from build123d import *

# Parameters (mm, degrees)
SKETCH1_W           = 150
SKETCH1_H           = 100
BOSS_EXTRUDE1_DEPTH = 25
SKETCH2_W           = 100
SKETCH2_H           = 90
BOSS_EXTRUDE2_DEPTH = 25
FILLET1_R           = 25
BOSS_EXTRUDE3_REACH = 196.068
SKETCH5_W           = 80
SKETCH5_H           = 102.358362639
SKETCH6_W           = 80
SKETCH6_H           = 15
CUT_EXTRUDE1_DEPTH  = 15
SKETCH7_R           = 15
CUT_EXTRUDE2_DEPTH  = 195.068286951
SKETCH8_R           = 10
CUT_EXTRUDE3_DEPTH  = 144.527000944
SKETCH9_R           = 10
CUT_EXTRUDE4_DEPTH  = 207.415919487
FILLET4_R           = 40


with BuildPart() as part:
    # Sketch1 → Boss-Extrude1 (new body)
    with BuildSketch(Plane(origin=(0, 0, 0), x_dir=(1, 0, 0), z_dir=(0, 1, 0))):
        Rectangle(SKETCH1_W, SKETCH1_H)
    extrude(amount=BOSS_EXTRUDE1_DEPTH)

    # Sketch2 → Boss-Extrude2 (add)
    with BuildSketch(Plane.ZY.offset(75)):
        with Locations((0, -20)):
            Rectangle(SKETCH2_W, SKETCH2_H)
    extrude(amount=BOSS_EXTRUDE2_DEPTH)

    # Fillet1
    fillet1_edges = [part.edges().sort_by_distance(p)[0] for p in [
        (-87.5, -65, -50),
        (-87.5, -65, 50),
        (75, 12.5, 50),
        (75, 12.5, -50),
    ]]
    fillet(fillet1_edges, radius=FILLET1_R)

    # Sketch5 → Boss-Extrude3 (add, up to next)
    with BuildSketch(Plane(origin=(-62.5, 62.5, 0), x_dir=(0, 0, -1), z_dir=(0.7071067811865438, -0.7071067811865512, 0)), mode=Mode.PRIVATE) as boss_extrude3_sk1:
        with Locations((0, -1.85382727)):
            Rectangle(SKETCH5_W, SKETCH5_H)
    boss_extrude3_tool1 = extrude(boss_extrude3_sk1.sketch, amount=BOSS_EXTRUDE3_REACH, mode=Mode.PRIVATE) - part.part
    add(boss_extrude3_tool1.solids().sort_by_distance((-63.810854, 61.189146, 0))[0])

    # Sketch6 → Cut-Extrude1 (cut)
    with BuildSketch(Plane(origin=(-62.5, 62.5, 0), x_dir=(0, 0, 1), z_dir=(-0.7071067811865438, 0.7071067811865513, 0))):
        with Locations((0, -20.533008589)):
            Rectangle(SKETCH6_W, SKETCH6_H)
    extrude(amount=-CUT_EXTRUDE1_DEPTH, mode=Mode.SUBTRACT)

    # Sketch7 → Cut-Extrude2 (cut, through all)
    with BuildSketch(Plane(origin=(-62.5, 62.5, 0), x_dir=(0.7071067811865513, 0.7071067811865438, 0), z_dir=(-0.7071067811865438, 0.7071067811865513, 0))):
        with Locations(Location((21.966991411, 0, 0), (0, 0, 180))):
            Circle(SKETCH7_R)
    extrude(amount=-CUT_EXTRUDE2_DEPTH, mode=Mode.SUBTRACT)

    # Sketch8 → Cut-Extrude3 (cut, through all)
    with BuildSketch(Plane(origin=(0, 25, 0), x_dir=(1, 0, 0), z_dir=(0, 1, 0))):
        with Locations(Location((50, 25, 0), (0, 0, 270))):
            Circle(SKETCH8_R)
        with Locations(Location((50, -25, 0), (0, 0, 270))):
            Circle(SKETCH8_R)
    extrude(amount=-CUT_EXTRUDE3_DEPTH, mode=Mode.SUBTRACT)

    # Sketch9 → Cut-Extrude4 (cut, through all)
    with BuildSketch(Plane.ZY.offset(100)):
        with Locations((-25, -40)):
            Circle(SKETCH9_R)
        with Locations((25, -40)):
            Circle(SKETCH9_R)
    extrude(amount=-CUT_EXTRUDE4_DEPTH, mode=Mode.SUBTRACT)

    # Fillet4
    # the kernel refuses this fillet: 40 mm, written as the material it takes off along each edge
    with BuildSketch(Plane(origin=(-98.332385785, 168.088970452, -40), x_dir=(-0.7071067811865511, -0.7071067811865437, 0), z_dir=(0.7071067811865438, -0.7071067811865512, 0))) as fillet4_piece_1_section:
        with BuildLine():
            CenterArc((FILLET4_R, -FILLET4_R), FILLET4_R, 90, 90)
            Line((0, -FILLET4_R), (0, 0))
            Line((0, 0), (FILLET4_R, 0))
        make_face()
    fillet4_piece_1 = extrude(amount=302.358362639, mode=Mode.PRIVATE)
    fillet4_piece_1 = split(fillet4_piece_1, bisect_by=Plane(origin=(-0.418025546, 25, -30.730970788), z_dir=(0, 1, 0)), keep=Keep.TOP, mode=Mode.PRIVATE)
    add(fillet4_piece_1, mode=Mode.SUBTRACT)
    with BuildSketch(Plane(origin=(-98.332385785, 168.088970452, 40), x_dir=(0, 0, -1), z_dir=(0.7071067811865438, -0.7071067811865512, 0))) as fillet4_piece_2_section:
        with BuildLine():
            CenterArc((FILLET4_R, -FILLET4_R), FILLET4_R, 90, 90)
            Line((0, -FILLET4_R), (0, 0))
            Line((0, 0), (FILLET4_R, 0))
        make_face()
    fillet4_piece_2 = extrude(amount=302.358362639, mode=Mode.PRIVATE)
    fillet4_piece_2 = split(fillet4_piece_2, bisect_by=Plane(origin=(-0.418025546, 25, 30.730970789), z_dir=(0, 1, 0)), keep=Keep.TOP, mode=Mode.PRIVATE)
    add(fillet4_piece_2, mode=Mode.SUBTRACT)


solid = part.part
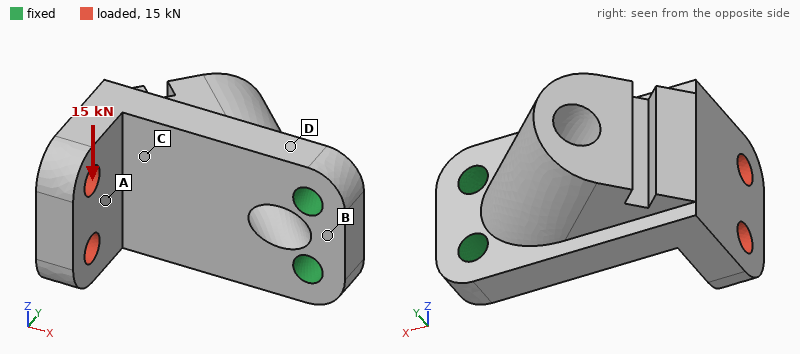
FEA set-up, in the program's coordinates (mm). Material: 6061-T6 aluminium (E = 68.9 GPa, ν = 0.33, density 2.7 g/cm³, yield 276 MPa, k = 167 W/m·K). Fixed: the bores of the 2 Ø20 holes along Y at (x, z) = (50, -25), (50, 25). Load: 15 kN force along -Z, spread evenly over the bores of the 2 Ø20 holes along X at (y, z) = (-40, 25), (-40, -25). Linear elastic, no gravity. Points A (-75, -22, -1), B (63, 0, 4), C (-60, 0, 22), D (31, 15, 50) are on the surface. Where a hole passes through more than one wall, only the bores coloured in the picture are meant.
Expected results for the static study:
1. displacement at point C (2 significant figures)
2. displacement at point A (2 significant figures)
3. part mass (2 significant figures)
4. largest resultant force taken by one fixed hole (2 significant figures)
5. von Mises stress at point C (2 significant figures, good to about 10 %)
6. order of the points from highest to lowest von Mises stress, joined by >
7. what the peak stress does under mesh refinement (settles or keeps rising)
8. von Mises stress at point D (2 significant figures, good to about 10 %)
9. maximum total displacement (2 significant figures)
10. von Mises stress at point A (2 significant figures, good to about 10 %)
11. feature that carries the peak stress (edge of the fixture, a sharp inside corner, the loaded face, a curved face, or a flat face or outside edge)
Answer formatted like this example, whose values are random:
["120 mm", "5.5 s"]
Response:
["0.17 mm", "0.26 mm", "2.2 kg", "30 kN", "37 MPa", "D > C > A > B", "keeps rising", "61 MPa", "0.42 mm", "16 MPa", "edge of the fixture"]
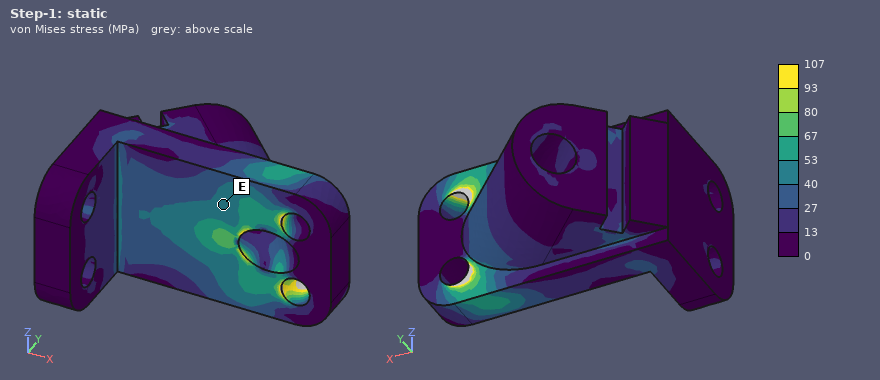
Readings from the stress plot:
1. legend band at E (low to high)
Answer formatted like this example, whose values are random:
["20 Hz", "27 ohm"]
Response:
["40 to 53 MPa"]
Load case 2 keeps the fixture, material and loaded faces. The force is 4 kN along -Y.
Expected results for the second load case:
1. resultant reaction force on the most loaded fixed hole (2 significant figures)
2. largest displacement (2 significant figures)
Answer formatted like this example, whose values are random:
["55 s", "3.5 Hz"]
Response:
["2.6 kN", "0.28 mm"]
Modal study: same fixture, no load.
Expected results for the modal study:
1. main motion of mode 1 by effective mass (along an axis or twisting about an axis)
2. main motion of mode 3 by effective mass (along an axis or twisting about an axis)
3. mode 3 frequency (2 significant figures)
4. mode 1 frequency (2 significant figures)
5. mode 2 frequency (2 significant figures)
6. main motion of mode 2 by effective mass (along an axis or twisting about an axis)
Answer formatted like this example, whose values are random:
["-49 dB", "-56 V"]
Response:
["along Y", "along Z", "2200 Hz", "650 Hz", "1400 Hz", "along Z"]
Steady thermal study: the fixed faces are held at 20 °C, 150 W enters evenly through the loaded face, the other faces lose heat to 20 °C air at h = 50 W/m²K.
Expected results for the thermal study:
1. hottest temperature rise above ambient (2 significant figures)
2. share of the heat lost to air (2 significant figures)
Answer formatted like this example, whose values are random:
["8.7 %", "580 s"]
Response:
["41 K", "43 %"]
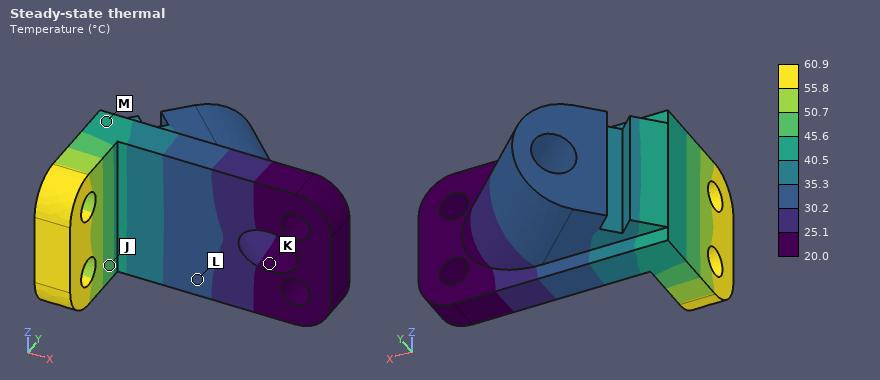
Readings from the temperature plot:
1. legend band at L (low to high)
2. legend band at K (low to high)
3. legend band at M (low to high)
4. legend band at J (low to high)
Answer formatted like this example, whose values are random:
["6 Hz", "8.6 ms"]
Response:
["30.2 to 35.3 °C", "20.0 to 25.1 °C", "40.5 to 45.6 °C", "45.6 to 50.7 °C"]
